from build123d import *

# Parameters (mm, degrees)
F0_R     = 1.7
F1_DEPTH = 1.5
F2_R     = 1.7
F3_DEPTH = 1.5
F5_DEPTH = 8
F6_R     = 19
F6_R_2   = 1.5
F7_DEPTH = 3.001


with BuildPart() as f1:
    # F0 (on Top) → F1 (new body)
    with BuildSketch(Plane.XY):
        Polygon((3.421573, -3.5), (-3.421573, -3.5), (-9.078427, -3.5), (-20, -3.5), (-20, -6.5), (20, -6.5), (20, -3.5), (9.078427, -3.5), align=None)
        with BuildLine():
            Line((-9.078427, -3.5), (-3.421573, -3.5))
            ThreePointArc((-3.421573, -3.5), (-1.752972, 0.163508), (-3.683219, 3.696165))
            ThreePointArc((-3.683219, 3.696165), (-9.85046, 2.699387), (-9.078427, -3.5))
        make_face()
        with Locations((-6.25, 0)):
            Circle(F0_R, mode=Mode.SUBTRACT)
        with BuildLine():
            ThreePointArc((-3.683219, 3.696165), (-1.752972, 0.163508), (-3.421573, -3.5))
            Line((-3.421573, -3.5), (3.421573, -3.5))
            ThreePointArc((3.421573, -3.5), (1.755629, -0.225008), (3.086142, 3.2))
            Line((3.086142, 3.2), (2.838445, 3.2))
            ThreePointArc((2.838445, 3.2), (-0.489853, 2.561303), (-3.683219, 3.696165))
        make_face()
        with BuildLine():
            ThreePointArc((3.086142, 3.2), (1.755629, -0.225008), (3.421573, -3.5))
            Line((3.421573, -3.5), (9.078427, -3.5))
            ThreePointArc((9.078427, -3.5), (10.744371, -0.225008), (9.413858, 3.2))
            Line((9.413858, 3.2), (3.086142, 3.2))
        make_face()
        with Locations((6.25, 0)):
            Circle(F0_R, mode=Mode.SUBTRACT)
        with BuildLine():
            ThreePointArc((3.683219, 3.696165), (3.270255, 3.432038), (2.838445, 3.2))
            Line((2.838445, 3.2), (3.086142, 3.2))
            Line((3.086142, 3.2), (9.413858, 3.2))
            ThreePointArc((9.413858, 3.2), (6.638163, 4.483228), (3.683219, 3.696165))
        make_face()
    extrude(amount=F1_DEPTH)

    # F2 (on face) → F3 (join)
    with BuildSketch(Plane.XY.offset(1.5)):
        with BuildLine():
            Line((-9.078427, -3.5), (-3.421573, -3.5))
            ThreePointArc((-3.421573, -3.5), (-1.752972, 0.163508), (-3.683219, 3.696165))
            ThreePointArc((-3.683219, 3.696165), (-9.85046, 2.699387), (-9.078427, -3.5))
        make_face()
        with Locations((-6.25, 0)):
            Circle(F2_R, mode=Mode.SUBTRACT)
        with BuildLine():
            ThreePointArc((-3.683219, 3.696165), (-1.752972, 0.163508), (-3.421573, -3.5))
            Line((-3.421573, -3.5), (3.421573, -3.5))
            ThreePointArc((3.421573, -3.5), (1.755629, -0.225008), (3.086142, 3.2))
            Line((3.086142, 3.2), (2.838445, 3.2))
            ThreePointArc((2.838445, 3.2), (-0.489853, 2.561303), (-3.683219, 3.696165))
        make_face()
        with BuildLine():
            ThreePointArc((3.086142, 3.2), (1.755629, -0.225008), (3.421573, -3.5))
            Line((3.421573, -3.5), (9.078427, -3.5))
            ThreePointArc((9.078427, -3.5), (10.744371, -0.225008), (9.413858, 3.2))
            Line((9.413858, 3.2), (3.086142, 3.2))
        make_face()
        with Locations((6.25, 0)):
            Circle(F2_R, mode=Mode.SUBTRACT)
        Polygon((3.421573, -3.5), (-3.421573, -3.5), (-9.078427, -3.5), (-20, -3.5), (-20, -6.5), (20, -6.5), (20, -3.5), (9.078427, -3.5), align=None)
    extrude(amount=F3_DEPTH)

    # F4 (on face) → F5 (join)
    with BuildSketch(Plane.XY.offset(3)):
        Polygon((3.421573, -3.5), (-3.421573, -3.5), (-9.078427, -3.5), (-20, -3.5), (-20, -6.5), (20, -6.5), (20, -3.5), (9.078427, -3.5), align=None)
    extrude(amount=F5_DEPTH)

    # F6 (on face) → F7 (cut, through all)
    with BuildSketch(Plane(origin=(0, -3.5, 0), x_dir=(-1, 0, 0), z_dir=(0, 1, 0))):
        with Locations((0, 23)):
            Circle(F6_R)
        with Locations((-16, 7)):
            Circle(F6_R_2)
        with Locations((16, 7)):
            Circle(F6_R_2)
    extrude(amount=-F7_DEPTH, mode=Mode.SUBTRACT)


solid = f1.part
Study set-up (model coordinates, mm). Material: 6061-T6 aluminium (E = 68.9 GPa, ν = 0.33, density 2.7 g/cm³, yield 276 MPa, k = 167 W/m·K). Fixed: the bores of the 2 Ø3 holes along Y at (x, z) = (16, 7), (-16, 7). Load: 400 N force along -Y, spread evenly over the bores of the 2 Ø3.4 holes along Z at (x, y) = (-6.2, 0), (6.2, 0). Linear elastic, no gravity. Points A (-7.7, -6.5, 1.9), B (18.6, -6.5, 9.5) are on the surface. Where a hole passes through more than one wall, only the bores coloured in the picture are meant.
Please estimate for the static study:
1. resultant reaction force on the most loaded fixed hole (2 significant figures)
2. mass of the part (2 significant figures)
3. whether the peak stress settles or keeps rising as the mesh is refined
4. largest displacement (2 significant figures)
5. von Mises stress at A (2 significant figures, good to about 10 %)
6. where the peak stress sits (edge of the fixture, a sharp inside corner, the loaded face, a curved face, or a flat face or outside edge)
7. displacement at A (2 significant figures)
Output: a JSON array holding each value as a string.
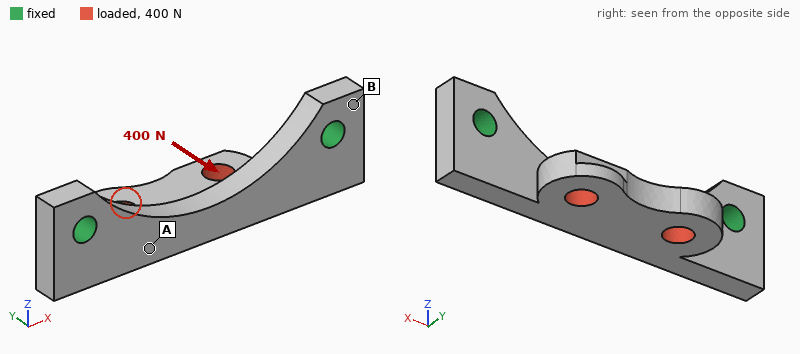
["200 N", "3.3 g", "keeps rising", "50 µm", "43 MPa", "edge of the fixture", "26 µm"]
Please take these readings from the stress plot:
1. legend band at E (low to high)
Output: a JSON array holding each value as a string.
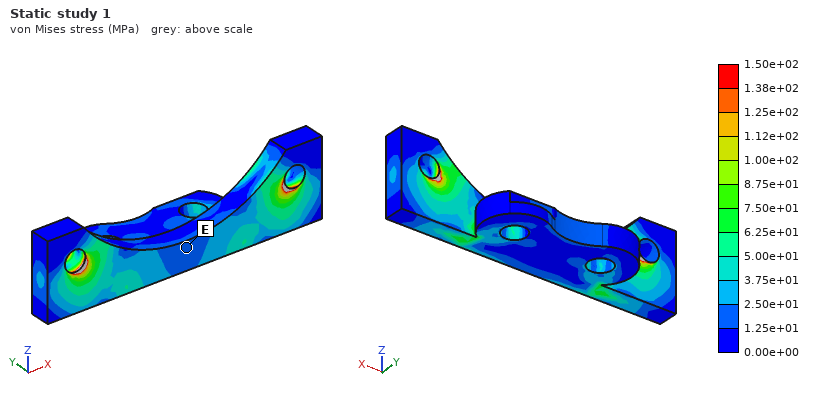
["1.25e+01 to 2.50e+01 MPa"]
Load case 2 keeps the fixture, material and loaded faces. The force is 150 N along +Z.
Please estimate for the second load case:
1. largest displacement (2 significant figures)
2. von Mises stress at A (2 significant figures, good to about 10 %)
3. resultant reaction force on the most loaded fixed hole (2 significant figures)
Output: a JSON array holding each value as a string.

["38 µm", "25 MPa", "110 N"]
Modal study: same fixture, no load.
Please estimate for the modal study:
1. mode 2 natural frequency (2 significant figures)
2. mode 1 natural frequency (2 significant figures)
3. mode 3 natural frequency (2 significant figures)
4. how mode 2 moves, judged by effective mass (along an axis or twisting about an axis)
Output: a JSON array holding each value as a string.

["18 kHz", "11 kHz", "22 kHz", "along Y"]
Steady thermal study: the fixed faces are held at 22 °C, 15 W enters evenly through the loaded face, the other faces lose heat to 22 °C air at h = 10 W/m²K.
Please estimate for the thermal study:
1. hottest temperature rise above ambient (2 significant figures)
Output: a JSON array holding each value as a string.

["31 K"]
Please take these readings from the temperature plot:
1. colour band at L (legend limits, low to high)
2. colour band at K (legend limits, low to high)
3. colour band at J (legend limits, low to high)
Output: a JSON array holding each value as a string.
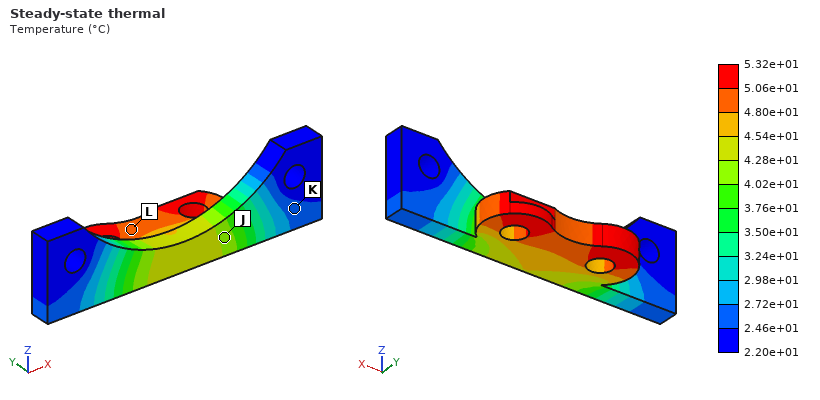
["4.80e+01 to 5.06e+01 °C", "2.46e+01 to 2.72e+01 °C", "4.02e+01 to 4.28e+01 °C"]
